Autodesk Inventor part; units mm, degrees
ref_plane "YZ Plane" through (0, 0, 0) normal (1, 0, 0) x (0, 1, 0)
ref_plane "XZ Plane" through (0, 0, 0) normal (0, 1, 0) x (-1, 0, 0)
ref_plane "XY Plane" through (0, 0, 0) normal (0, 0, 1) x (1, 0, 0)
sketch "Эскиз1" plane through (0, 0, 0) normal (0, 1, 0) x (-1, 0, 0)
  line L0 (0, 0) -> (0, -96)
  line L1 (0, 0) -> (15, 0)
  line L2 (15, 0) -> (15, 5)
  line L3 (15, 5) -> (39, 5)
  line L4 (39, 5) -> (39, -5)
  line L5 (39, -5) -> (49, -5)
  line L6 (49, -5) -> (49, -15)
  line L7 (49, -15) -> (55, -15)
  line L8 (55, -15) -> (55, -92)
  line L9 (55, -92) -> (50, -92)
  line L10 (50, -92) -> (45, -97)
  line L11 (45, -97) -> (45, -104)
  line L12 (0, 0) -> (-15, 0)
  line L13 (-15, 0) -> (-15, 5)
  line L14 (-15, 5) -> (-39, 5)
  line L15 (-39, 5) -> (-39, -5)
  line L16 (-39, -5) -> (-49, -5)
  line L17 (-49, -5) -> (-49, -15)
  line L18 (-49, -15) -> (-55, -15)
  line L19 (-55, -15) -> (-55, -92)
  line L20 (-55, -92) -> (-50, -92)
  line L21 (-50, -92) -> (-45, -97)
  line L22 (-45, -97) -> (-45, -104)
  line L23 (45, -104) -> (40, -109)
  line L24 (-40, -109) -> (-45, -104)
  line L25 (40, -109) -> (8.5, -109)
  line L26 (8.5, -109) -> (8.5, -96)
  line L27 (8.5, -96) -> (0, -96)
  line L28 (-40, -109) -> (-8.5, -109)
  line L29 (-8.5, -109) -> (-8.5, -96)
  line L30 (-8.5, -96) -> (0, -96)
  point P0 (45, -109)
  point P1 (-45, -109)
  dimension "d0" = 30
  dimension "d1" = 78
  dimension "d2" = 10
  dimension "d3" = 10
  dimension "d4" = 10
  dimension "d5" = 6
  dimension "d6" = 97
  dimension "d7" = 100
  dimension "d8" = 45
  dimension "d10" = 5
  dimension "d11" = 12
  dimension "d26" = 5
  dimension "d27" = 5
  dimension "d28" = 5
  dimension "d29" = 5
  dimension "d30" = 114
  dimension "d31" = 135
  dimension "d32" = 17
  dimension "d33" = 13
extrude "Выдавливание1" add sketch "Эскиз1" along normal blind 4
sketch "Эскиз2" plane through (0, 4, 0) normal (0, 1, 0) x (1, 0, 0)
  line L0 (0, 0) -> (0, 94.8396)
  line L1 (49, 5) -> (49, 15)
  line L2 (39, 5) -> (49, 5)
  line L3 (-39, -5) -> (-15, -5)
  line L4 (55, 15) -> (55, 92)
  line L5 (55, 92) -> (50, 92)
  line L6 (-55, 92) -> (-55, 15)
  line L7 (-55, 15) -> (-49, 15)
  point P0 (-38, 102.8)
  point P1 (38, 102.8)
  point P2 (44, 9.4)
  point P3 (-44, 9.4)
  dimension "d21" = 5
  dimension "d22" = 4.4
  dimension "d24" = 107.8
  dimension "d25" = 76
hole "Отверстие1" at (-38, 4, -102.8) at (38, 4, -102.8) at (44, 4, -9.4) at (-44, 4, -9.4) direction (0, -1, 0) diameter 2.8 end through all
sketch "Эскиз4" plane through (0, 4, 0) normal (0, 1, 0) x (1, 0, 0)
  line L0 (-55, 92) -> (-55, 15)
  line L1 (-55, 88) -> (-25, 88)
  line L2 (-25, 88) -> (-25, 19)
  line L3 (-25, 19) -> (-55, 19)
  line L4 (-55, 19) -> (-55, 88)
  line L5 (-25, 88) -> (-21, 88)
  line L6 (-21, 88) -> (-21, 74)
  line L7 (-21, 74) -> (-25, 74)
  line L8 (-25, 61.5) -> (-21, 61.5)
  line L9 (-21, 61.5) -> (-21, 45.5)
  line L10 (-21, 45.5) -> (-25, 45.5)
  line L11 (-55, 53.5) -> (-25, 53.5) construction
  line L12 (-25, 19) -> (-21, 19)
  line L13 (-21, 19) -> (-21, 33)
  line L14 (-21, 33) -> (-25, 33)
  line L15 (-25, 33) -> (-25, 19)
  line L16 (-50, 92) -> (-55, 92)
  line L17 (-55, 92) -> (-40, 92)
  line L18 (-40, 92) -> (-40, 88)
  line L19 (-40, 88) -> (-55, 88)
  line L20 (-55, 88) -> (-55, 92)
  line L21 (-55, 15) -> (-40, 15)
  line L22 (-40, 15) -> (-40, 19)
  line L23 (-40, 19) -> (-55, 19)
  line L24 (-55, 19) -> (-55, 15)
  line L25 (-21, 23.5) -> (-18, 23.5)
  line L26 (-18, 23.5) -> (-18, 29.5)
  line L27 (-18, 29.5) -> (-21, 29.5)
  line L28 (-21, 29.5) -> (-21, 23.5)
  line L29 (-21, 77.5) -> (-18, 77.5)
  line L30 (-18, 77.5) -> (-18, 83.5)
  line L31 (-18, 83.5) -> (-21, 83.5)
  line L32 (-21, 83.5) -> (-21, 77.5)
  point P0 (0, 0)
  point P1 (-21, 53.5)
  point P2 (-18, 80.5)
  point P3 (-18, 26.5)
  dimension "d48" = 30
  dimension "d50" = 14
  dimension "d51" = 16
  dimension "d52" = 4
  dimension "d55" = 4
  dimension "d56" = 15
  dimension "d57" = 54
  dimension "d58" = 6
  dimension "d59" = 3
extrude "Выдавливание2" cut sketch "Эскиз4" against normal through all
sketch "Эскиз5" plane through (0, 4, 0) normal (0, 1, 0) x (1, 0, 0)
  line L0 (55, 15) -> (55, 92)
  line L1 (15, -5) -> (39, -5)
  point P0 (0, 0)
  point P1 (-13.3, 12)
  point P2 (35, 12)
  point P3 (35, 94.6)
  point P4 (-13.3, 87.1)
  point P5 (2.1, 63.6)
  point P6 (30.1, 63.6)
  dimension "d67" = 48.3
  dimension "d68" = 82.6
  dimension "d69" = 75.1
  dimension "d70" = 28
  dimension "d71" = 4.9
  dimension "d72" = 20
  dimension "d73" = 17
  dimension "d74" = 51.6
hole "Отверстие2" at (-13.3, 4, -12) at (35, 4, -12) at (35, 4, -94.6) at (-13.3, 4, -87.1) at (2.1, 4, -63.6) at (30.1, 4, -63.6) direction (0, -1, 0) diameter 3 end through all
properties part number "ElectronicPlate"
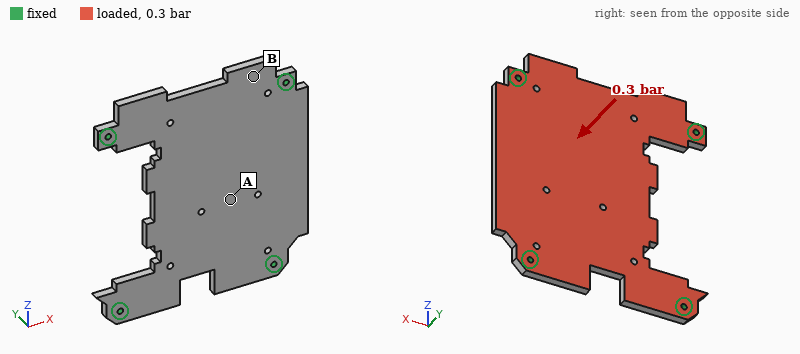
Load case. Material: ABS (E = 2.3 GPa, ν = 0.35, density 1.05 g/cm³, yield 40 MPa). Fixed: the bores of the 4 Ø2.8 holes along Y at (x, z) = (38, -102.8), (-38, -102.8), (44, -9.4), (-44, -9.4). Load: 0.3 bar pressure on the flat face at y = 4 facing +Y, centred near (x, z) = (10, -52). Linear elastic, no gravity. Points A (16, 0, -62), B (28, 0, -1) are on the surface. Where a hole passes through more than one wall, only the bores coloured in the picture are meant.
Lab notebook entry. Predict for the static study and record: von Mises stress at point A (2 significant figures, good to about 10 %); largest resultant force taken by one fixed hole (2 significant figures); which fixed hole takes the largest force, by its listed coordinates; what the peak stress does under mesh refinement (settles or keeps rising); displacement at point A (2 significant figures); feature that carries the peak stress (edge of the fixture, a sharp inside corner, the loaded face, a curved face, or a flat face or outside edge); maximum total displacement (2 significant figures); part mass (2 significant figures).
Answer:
5.0 MPa
90 N
(44, -9.4)
keeps rising
1.2 mm
edge of the fixture
1.6 mm
37 g
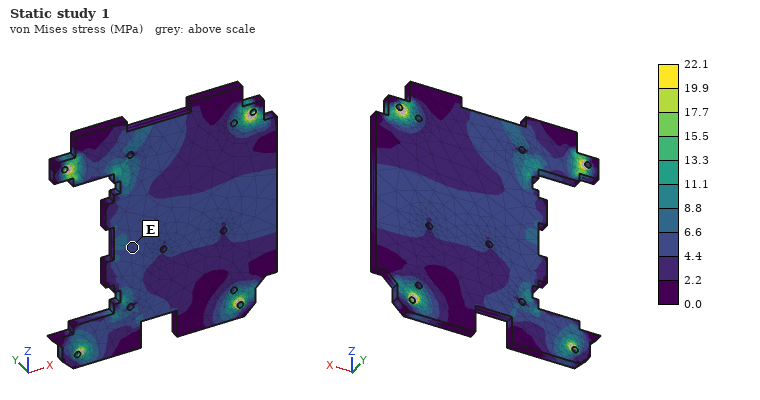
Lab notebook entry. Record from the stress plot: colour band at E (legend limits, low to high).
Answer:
4.4 to 6.6 MPa
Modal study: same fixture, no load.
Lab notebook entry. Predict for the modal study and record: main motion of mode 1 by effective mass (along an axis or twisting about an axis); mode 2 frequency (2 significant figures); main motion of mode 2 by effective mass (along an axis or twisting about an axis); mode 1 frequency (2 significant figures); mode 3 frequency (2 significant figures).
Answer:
along Y
660 Hz
twisting about Z
420 Hz
770 Hz
